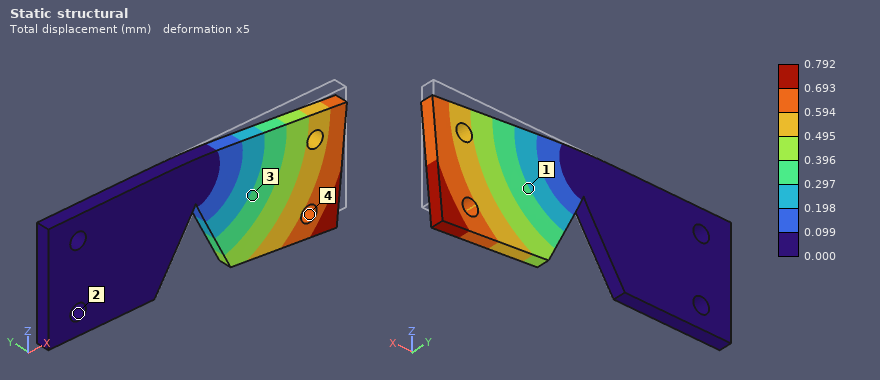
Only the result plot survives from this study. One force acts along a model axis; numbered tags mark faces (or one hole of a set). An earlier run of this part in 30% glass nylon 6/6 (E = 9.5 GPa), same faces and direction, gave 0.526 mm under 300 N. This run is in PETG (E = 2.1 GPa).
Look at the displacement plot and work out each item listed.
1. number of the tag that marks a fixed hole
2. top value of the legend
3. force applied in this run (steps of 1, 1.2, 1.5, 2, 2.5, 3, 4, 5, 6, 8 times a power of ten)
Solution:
2
0.792 mm
100 N
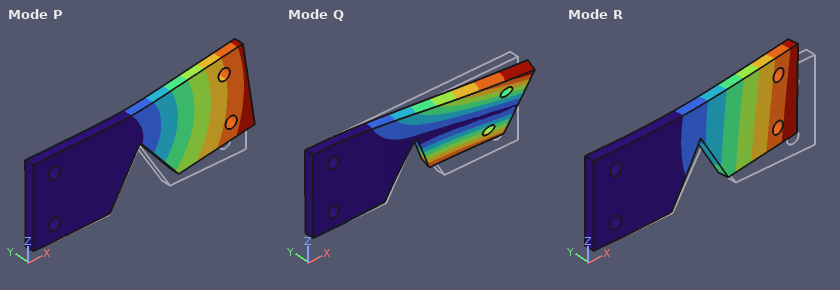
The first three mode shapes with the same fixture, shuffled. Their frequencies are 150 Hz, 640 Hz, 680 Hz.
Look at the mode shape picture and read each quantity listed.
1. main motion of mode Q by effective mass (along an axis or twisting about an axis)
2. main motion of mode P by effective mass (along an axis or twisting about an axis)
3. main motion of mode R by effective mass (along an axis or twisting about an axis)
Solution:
twisting about X
along Z
along Y
